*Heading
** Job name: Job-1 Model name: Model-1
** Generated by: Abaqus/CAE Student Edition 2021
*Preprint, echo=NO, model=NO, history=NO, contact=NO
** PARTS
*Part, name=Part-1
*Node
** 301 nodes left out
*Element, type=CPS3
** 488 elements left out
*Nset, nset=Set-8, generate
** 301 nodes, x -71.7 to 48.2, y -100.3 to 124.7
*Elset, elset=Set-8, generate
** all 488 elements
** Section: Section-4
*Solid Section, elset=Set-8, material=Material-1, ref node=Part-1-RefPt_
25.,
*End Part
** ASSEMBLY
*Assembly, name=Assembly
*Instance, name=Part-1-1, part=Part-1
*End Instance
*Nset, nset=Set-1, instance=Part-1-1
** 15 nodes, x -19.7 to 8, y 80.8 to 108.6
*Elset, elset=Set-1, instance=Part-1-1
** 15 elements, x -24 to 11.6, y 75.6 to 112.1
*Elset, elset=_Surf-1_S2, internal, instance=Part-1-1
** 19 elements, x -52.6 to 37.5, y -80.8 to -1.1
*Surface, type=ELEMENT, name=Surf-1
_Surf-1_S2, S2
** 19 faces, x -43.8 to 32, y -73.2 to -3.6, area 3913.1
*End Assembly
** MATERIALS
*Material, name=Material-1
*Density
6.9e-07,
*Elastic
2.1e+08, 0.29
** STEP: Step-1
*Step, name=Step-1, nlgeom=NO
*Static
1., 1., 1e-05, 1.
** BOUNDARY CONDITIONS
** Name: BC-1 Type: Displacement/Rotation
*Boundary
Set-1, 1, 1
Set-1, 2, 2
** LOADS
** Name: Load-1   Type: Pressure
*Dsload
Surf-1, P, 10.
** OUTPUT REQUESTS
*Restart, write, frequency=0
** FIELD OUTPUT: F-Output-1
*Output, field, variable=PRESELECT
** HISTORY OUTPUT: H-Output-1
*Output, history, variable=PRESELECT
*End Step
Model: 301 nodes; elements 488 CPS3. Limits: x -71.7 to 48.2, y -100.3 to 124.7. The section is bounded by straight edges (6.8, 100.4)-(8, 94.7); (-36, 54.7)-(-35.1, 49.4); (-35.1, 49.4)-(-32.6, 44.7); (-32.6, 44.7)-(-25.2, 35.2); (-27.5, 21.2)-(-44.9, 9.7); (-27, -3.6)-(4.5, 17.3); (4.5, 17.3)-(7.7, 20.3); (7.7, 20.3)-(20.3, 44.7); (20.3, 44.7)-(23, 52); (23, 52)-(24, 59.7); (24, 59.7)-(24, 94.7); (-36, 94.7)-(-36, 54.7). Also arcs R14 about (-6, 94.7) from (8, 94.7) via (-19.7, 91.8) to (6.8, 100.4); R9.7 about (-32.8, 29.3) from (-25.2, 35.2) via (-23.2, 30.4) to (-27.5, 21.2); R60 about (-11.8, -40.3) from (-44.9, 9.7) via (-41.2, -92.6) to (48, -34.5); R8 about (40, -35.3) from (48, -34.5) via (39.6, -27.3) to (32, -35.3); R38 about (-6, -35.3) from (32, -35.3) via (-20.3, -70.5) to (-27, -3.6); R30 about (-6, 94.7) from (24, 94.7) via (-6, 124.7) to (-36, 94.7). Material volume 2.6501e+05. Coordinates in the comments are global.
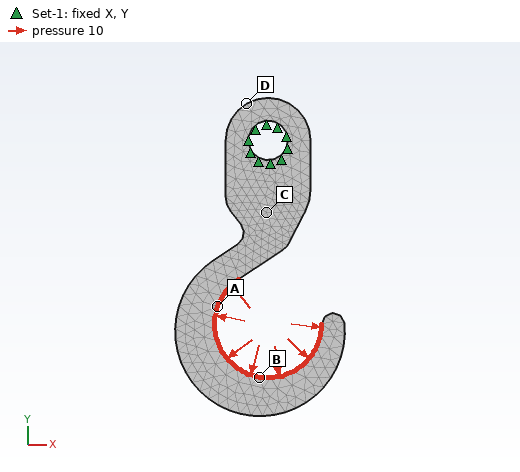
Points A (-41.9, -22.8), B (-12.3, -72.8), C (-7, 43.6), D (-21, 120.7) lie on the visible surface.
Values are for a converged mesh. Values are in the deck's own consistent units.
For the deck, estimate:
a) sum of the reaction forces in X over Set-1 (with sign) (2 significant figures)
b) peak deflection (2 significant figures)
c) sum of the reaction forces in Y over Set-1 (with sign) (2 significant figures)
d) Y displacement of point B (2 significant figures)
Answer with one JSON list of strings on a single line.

["7900", "0.0017", "15000", "-4.7e-04"]
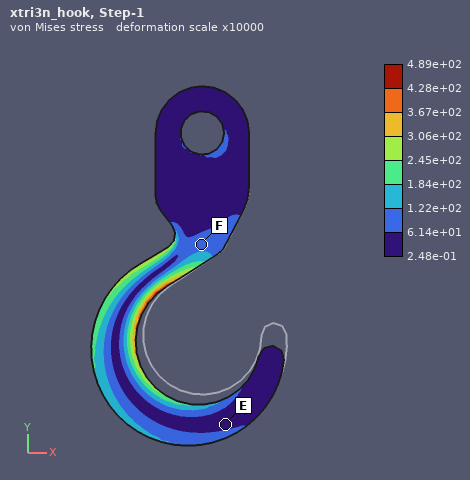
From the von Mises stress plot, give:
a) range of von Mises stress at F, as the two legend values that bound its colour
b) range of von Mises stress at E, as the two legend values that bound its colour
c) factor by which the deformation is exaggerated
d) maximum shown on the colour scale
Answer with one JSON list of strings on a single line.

["6.14e+01 to 1.22e+02", "2.48e-01 to 6.14e+01", "10000", "4.89e+02"]
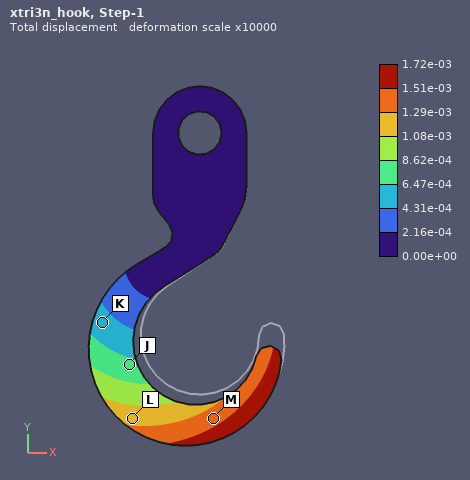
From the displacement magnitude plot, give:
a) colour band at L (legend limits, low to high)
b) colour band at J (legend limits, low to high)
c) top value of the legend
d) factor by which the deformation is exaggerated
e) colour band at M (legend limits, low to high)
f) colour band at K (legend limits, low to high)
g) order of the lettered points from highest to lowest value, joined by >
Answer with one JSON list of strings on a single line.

["1.08e-03 to 1.29e-03", "6.47e-04 to 8.62e-04", "1.72e-03", "10000", "1.29e-03 to 1.51e-03", "4.31e-04 to 6.47e-04", "M > L > J > K"]
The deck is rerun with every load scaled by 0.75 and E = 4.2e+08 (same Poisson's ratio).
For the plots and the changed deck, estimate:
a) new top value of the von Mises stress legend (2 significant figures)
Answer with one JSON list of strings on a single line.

["370"]
